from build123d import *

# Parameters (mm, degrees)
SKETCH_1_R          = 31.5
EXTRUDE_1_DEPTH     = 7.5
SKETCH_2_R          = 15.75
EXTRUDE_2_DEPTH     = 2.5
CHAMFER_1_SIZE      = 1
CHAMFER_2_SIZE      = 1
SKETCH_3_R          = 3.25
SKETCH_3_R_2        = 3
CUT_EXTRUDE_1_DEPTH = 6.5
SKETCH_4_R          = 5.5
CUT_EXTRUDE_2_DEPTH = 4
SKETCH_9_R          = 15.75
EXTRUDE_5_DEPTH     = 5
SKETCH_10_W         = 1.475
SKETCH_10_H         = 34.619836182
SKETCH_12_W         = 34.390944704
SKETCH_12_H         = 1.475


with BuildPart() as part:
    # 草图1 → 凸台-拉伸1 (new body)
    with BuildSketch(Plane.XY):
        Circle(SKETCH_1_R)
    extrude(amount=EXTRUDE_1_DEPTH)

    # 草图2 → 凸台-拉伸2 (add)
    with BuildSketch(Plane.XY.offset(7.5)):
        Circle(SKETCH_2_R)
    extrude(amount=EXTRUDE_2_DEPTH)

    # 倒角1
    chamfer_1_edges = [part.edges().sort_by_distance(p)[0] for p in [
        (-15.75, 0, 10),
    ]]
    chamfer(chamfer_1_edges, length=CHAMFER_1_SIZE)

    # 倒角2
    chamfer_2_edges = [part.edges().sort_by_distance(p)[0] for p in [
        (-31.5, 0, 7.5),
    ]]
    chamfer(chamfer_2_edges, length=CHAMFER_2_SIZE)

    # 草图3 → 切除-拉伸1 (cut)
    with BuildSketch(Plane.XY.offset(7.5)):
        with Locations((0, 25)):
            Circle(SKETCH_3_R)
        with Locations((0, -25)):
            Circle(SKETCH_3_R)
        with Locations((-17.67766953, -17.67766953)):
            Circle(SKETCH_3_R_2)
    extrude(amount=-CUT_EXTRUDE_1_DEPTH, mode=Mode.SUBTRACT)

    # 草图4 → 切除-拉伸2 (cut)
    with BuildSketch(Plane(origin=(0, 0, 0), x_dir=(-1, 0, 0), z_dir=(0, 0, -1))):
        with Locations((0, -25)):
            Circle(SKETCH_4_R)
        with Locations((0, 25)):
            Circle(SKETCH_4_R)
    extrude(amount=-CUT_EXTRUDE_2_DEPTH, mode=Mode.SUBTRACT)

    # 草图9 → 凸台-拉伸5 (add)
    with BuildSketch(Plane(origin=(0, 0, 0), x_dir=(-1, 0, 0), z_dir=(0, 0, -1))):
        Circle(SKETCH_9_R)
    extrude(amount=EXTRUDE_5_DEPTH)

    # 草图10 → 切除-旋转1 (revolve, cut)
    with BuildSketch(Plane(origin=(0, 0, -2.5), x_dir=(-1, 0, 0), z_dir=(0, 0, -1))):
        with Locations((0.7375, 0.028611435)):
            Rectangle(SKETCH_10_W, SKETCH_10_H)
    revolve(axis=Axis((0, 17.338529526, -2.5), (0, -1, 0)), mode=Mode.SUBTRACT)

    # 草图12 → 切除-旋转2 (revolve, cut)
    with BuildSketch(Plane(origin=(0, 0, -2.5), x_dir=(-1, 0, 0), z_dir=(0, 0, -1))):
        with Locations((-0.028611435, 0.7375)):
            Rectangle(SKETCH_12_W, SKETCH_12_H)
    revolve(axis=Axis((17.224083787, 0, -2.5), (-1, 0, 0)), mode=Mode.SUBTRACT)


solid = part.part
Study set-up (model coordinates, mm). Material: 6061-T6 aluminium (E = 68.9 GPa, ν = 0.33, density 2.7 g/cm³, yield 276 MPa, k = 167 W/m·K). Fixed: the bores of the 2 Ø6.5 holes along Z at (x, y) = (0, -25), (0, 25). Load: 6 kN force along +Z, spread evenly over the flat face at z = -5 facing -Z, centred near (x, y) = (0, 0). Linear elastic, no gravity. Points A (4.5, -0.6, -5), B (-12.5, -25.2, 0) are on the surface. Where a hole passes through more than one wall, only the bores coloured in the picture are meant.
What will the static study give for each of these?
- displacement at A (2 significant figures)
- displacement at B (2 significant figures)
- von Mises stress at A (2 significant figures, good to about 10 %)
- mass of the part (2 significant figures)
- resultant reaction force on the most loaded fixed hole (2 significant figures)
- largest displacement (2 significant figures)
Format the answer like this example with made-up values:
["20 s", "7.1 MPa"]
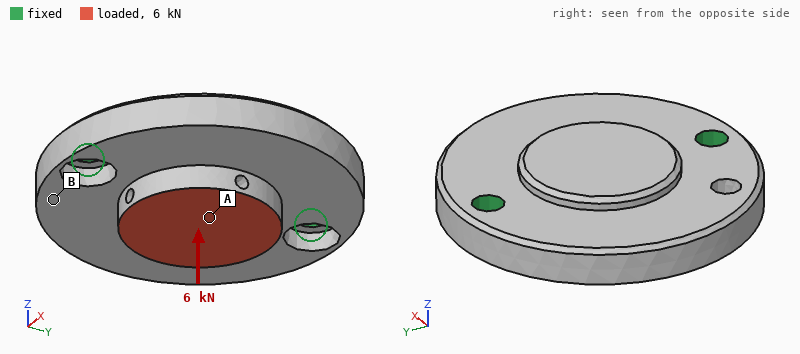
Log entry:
["34 µm", "14 µm", "53 MPa", "74 g", "3.5 kN", "47 µm"]
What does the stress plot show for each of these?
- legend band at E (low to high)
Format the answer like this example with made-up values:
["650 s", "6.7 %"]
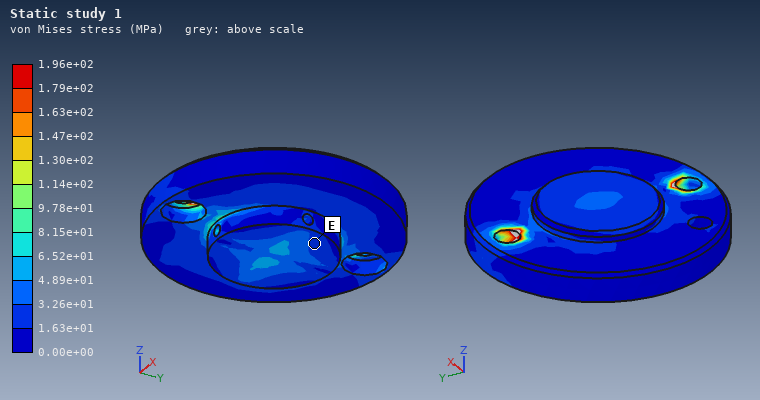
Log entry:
["1.63e+01 to 3.26e+01 MPa"]
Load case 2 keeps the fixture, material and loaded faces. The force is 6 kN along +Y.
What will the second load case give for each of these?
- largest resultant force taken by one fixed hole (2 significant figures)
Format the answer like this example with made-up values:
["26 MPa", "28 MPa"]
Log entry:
["3.3 kN"]
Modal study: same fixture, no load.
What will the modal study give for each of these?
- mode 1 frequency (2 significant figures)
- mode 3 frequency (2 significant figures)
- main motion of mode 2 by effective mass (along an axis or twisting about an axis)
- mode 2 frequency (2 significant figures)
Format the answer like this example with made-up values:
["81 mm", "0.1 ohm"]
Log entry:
["3400 Hz", "15 kHz", "along Z", "7600 Hz"]
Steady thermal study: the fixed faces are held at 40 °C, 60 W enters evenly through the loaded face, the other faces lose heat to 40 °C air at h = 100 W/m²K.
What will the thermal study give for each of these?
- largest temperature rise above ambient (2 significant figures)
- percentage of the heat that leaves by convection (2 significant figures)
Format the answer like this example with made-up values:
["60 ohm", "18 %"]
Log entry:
["19 K", "15 %"]
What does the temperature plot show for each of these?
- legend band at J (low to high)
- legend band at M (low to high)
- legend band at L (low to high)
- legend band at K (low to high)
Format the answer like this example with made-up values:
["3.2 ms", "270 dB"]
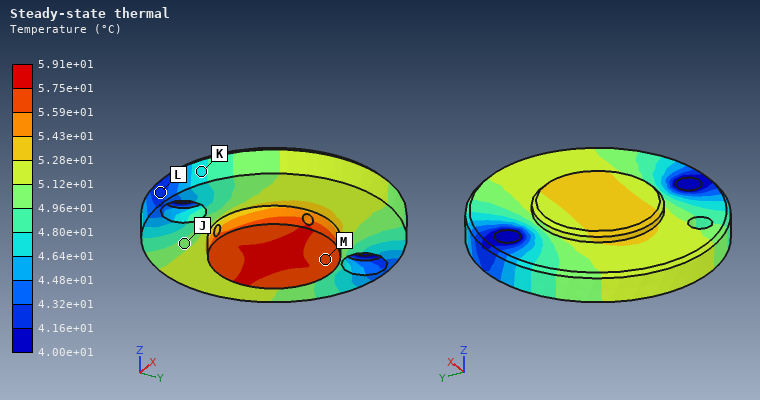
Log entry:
["4.96e+01 to 5.12e+01 °C", "5.59e+01 to 5.75e+01 °C", "4.16e+01 to 4.32e+01 °C", "4.64e+01 to 4.80e+01 °C"]
